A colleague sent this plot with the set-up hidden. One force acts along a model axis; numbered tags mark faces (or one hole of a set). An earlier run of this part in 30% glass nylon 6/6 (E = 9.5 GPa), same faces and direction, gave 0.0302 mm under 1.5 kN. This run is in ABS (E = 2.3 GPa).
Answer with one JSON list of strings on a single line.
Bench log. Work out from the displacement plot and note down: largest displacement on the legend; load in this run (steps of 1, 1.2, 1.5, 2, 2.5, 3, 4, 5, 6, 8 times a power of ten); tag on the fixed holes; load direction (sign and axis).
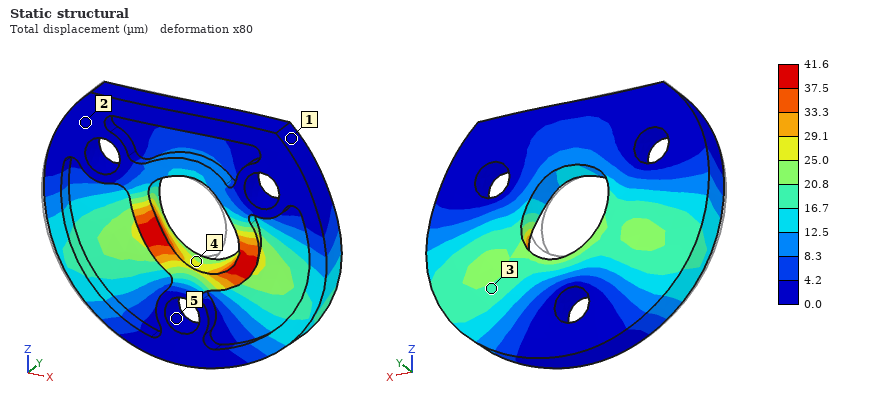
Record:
["41.6 µm", "500 N", "5", "+X"]
